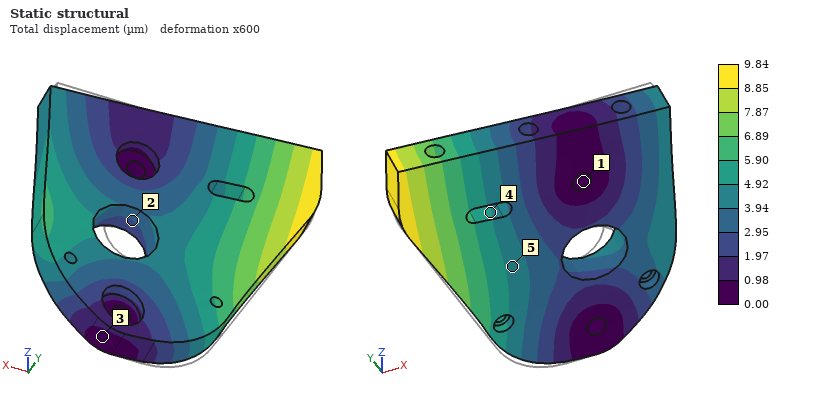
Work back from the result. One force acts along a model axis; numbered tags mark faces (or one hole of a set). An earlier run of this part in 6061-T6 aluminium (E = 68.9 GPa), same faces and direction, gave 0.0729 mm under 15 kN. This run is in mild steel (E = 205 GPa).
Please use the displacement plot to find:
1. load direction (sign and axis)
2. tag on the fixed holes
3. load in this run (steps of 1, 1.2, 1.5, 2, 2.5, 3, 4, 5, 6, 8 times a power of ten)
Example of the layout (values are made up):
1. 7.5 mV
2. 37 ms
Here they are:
1. +X
2. 1
3. 6 kN
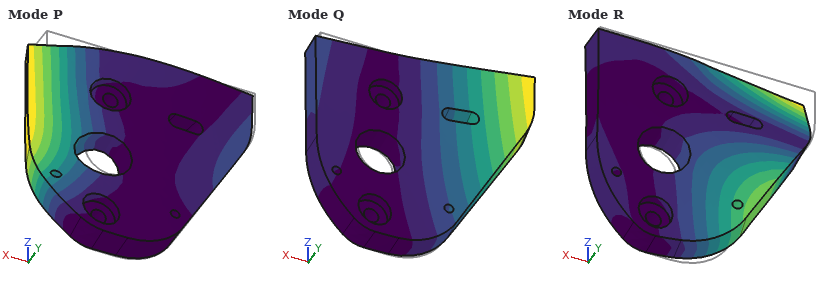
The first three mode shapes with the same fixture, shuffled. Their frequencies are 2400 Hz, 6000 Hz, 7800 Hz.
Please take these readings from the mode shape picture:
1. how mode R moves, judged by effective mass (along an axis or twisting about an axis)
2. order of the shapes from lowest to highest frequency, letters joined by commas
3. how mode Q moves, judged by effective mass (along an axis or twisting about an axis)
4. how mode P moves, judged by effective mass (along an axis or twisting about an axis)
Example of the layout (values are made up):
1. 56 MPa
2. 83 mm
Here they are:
1. twisting about X
2. Q, R, P
3. along Y
4. along Y
